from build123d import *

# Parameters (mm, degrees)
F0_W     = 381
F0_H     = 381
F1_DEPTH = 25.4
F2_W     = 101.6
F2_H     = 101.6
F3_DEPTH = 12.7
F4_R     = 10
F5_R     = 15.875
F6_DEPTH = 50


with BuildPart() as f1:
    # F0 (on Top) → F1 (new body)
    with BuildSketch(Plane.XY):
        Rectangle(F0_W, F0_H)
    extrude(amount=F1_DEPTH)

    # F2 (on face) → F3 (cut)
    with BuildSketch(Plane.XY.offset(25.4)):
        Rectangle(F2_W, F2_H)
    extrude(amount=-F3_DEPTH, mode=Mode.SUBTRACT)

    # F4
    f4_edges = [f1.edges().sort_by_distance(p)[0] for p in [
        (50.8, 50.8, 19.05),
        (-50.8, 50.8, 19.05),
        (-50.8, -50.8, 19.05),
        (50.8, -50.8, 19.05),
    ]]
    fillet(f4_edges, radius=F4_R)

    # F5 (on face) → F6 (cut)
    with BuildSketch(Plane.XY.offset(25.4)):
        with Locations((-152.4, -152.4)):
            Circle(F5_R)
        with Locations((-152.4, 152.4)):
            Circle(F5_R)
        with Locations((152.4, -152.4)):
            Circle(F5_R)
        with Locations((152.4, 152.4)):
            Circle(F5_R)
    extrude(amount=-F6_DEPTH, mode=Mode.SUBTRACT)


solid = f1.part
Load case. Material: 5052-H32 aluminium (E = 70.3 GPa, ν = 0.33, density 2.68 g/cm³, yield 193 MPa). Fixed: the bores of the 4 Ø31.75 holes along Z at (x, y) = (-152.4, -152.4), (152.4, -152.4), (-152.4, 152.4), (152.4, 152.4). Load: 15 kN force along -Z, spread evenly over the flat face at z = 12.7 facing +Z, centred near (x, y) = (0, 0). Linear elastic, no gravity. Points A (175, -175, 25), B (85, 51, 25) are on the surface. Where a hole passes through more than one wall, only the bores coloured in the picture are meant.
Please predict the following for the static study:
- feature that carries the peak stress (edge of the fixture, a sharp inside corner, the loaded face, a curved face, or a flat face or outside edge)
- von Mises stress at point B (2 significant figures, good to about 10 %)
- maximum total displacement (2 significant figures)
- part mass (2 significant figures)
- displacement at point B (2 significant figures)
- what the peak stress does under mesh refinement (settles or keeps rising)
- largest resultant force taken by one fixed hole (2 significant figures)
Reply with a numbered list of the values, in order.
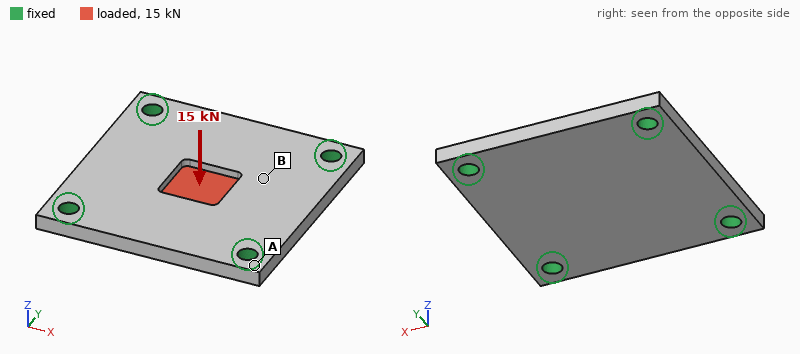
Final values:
1. edge of the fixture
2. 14 MPa
3. 0.24 mm
4. 9.3 kg
5. 0.11 mm
6. keeps rising
7. 4.8 kN
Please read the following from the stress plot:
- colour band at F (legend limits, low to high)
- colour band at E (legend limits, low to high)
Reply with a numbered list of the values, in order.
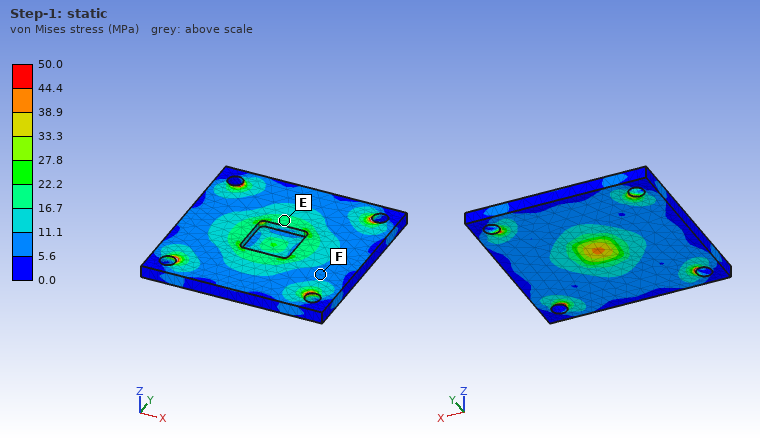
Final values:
1. 5.6 to 11.1 MPa
2. 16.7 to 22.2 MPa
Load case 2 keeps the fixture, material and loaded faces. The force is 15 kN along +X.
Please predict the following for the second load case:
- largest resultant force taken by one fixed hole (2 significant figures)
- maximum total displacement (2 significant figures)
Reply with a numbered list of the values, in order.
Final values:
1. 4.2 kN
2. 9.7 µm
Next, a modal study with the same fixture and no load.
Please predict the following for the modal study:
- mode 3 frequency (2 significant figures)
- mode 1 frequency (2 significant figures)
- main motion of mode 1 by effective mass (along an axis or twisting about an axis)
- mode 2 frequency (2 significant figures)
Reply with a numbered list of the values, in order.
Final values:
1. 1600 Hz
2. 1000 Hz
3. along Z
4. 1600 Hz
